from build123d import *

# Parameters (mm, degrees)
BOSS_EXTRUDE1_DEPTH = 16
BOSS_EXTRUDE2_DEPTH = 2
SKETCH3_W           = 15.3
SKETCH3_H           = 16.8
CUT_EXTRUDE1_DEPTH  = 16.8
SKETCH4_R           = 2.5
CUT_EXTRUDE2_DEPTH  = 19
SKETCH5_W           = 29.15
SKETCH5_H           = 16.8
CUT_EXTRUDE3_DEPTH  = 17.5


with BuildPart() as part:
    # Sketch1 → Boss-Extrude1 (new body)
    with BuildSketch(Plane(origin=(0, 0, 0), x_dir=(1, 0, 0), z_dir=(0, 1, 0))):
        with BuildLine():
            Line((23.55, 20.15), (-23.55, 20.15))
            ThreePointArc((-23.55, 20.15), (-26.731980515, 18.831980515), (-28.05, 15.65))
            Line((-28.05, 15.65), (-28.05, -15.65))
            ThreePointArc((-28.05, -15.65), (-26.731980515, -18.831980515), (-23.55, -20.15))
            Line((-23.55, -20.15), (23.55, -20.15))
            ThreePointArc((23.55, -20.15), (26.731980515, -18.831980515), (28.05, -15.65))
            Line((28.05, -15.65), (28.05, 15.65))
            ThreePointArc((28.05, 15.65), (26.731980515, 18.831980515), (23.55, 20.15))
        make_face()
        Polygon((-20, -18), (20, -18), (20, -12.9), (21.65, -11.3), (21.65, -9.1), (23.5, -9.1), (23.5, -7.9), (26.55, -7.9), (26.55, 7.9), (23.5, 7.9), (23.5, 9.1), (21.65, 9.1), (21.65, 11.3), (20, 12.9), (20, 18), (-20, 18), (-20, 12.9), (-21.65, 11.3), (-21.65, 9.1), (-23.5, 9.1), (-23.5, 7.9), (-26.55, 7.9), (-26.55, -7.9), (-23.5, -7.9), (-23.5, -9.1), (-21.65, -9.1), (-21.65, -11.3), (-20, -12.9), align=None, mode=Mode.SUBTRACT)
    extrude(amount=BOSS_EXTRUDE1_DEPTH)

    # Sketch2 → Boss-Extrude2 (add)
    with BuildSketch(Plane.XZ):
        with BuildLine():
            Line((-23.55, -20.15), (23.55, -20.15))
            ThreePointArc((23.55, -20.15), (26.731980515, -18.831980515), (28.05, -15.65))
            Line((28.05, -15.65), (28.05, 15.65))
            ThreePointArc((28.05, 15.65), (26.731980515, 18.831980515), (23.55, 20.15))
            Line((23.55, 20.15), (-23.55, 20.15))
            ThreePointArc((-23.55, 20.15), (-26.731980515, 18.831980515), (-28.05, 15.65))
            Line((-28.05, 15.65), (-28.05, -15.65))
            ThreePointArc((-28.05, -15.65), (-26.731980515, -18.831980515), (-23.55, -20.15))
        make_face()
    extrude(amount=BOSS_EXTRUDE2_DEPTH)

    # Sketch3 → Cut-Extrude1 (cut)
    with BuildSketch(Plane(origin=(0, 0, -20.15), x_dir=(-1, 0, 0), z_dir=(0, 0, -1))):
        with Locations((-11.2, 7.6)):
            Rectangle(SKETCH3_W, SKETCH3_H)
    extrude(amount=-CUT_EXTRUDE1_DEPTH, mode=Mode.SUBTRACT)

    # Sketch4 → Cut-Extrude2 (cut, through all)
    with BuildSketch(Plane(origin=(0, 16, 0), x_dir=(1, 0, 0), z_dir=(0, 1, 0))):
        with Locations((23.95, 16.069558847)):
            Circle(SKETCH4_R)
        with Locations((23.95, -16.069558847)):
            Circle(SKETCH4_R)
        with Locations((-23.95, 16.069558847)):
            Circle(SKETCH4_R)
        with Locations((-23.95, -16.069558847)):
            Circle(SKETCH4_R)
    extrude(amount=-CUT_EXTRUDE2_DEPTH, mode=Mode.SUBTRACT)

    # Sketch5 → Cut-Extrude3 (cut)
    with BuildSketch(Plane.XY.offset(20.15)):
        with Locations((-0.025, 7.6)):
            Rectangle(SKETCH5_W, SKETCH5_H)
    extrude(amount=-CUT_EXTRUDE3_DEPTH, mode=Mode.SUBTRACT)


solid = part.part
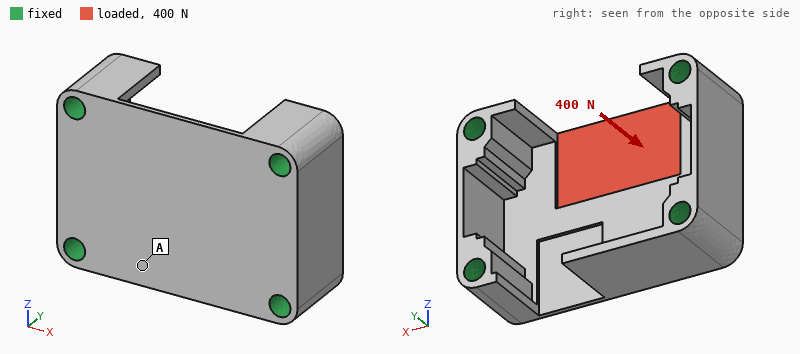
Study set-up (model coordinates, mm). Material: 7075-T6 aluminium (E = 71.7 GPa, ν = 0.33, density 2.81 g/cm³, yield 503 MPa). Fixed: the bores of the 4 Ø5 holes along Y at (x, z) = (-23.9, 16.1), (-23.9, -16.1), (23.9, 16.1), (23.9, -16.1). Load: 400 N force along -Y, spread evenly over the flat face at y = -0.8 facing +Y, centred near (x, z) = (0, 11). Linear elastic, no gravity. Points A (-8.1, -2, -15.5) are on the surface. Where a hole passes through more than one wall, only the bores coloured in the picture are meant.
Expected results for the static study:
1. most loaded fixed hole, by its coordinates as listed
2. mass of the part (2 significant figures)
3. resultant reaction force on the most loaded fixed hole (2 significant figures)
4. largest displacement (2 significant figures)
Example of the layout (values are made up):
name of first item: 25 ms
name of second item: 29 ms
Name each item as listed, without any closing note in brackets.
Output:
most loaded fixed hole, by its coordinates as listed: (23.9, 16.1)
mass of the part: 28 g
resultant reaction force on the most loaded fixed hole: 270 N
largest displacement: 0.18 mm
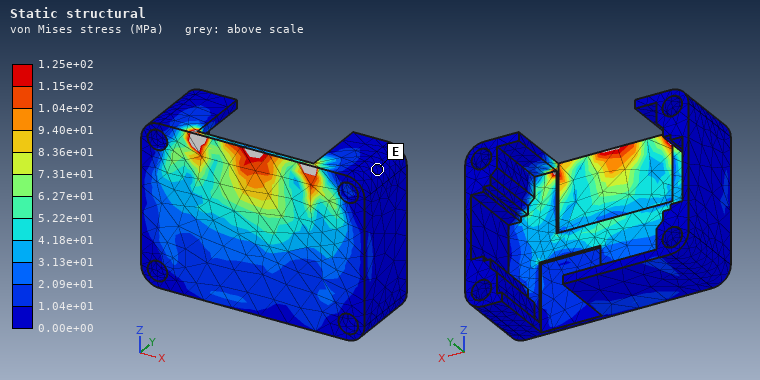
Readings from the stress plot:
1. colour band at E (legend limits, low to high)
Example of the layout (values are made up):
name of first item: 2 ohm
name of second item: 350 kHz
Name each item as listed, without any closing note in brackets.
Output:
colour band at E: 0.00e+00 to 1.04e+01 MPa
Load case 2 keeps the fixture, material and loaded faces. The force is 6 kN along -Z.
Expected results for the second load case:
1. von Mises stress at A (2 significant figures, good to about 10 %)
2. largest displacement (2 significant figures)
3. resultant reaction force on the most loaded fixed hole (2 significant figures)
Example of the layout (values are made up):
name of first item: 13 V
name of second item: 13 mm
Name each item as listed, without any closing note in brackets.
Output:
von Mises stress at A: 37 MPa
largest displacement: 0.21 mm
resultant reaction force on the most loaded fixed hole: 1.9 kN
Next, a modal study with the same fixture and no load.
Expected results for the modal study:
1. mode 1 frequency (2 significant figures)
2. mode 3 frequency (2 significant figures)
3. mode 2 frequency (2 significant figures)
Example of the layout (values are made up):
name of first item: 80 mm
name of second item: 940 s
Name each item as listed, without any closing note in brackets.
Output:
mode 1 frequency: 5700 Hz
mode 3 frequency: 9300 Hz
mode 2 frequency: 7400 Hz
